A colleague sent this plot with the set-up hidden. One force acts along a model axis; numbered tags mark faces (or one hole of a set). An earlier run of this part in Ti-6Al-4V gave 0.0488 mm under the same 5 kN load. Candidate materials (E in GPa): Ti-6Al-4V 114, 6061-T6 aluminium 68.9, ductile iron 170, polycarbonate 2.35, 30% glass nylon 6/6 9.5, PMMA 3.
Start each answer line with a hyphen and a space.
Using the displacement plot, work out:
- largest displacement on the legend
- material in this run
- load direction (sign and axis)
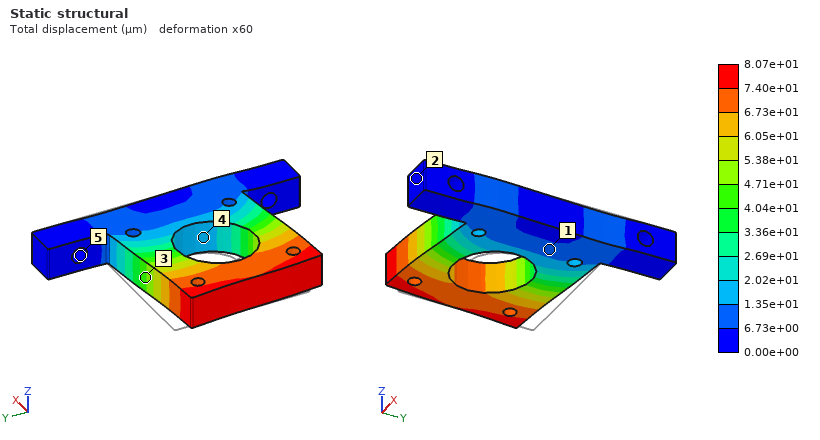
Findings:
- 8.07e+01 µm
- 6061-T6 aluminium
- -Y
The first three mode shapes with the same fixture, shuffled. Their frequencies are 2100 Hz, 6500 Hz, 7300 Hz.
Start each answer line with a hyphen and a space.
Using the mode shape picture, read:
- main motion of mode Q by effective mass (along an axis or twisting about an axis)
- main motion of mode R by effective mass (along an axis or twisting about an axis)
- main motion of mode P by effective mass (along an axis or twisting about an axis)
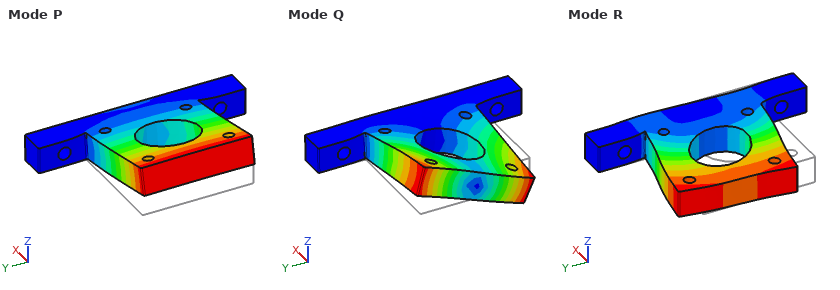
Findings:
- twisting about X
- along Y
- along Z
